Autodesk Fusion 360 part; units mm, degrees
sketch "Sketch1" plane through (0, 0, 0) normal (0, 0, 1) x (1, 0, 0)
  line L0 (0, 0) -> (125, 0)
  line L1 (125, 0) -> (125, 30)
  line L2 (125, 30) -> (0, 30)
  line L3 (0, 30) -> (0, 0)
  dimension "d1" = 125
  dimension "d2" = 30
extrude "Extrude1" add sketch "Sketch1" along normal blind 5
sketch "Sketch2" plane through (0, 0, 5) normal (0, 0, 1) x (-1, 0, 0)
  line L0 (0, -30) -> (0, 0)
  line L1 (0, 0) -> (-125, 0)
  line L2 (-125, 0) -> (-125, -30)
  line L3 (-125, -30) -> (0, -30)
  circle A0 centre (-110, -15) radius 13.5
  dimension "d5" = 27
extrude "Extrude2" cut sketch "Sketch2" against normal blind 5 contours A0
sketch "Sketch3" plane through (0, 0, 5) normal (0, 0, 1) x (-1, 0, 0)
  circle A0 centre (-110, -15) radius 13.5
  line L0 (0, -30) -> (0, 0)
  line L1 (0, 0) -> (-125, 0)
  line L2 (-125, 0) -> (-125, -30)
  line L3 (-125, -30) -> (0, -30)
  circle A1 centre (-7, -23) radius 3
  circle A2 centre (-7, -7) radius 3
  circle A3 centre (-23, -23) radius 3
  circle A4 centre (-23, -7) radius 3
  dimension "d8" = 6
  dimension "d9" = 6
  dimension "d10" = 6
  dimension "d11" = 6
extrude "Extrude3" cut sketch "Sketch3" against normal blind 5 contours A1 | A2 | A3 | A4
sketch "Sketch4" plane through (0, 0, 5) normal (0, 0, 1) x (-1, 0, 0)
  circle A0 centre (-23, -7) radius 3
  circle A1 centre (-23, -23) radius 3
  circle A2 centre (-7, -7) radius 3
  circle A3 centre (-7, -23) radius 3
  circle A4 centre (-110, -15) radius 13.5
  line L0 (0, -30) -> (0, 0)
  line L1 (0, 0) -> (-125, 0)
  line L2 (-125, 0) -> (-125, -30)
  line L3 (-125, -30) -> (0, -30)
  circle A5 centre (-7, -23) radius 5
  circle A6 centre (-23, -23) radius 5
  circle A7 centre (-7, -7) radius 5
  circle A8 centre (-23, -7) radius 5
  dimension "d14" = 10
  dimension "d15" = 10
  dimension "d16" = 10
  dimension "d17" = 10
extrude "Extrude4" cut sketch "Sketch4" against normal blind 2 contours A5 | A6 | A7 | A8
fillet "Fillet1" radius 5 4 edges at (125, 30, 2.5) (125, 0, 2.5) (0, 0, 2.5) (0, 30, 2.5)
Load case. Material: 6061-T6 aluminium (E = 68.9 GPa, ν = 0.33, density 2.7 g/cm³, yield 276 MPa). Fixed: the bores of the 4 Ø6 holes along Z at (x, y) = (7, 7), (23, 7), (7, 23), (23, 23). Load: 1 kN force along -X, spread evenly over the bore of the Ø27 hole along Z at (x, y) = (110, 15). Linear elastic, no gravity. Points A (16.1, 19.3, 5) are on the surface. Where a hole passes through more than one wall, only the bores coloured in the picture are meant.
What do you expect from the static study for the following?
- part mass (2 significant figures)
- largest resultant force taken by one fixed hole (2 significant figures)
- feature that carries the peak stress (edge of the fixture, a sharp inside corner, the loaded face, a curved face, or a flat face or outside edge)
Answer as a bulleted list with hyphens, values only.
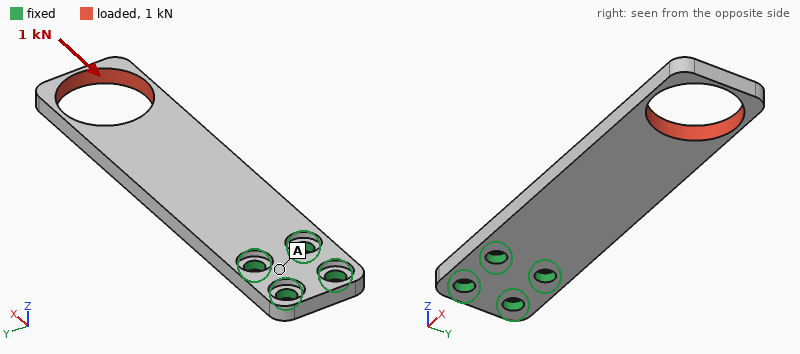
- 40 g
- 440 N
- the loaded face
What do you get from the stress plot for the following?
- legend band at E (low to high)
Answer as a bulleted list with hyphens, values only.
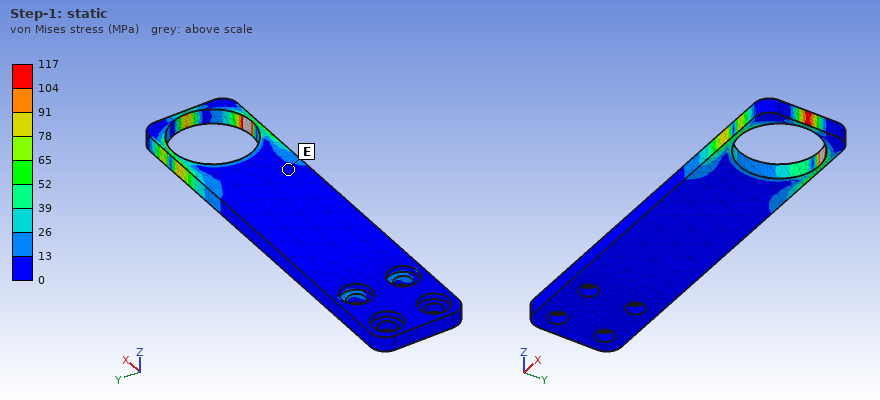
- 0 to 13 MPa
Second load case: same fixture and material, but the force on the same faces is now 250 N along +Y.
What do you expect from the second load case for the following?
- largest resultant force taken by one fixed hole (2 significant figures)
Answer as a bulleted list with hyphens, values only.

- 960 N
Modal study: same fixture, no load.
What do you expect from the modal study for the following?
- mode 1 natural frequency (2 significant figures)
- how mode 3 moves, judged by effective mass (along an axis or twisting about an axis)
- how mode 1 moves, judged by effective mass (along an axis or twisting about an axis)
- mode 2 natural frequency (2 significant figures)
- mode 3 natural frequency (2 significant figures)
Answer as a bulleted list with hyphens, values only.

- 520 Hz
- along Y
- along Z
- 2400 Hz
- 2600 Hz
